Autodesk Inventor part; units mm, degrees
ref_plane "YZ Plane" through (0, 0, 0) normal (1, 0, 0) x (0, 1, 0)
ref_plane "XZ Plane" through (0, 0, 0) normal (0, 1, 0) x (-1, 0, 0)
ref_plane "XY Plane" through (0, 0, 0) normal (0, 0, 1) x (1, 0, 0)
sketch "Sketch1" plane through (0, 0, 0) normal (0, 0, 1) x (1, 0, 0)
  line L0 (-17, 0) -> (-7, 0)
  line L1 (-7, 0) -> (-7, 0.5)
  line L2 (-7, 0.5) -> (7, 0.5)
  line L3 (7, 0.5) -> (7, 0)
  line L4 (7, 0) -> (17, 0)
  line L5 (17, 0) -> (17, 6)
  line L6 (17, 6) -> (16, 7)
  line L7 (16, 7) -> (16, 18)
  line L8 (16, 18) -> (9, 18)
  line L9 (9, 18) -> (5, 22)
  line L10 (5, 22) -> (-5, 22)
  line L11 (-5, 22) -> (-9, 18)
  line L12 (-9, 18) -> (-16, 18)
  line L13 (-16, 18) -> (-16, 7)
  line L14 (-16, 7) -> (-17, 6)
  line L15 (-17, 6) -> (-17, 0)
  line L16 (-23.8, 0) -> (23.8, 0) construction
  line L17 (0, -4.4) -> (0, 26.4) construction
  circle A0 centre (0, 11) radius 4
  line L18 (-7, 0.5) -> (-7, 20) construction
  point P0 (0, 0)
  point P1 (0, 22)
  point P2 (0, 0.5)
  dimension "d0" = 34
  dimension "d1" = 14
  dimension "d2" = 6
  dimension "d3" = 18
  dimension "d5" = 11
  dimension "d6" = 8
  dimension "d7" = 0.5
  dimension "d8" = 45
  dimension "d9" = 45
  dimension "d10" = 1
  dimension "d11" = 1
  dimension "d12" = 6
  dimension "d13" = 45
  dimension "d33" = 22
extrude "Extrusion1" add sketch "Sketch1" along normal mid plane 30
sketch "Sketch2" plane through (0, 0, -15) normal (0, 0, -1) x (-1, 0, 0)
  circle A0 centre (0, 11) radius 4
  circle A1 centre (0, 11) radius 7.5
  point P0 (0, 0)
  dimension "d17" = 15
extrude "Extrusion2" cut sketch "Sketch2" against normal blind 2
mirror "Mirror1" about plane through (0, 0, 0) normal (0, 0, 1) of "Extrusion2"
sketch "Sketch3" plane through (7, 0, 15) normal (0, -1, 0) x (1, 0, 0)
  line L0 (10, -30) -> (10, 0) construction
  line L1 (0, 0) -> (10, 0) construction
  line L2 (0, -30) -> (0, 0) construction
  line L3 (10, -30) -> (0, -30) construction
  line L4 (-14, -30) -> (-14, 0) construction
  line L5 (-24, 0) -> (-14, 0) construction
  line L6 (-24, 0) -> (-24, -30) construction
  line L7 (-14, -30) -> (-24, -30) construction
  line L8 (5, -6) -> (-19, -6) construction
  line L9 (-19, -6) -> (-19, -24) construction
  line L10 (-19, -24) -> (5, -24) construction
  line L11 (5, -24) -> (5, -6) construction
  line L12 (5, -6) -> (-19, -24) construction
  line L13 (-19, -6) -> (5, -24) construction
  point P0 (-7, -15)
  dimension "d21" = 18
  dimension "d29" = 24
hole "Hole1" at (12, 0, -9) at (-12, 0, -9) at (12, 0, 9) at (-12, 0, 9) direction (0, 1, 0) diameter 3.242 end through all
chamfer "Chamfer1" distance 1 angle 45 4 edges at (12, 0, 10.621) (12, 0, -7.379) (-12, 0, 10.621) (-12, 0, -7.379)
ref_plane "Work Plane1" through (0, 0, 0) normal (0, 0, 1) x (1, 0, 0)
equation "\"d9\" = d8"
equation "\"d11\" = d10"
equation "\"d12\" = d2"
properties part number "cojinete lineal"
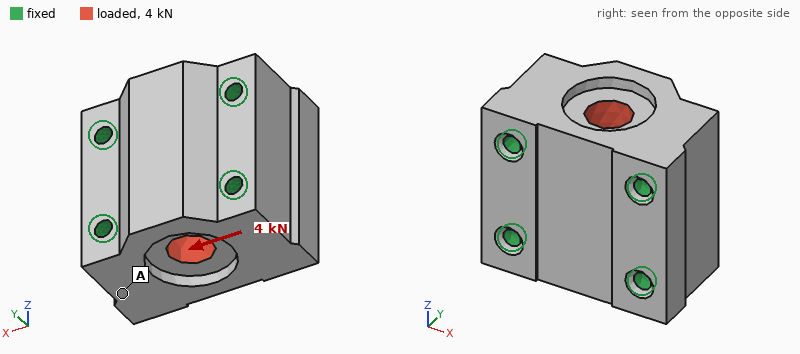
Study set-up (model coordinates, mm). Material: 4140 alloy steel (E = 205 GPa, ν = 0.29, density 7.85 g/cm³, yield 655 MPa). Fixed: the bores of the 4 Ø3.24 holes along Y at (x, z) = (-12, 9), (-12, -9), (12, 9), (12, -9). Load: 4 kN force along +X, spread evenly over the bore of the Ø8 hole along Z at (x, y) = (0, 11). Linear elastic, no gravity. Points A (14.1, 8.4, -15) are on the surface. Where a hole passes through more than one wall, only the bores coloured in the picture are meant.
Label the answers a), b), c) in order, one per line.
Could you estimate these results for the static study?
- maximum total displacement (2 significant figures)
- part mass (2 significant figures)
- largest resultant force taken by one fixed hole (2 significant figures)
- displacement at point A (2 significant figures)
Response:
a) 0.42 µm
b) 130 g
c) 1.0 kN
d) 0.065 µm
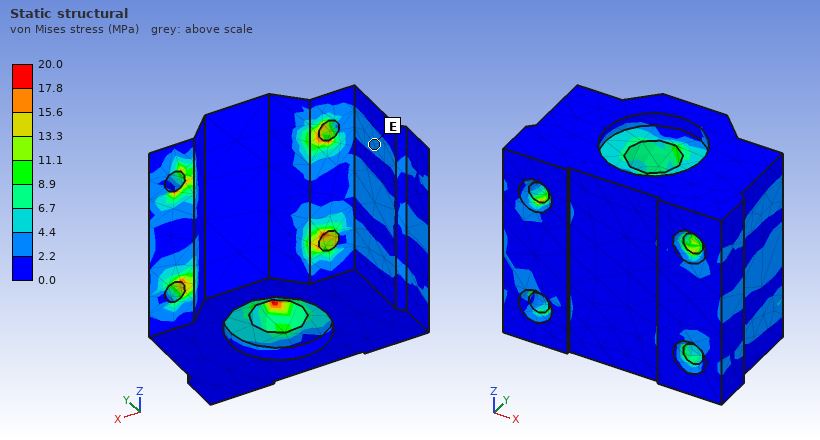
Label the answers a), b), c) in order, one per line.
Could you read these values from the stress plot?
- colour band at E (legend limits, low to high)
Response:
a) 2.2 to 4.4 MPa
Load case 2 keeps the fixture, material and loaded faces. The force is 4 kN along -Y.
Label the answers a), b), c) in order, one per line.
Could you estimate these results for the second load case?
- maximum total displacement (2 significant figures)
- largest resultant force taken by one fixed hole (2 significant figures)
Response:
a) 0.77 µm
b) 1.0 kN
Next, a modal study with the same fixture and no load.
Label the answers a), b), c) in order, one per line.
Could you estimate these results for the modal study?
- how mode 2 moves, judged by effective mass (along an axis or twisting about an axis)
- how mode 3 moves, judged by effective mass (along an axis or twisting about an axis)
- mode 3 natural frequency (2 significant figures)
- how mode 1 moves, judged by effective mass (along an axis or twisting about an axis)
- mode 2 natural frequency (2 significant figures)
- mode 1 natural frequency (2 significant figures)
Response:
a) along Y
b) along Z
c) 63 kHz
d) along Z
e) 54 kHz
f) 52 kHz
